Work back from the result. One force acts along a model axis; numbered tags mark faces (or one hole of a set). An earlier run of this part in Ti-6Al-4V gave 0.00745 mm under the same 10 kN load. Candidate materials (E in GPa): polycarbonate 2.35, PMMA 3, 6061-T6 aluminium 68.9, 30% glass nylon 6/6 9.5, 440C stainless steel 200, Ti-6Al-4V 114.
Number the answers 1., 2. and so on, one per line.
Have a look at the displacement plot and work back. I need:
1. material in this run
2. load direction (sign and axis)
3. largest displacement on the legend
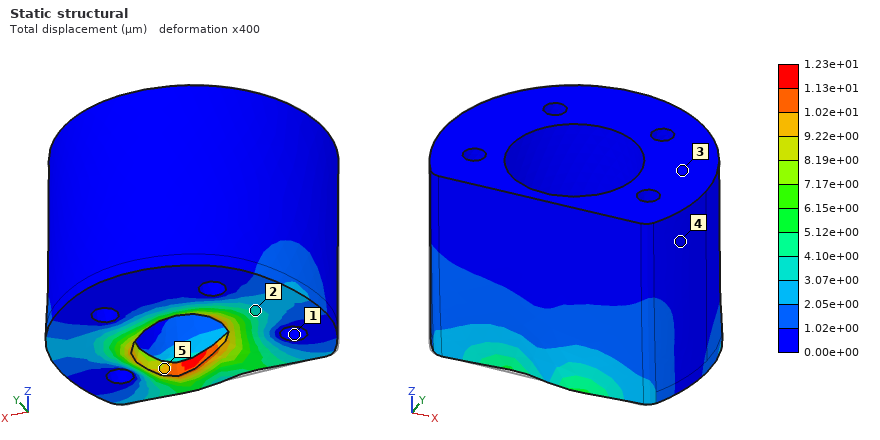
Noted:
1. 6061-T6 aluminium
2. +X
3. 1.23e+01 µm
